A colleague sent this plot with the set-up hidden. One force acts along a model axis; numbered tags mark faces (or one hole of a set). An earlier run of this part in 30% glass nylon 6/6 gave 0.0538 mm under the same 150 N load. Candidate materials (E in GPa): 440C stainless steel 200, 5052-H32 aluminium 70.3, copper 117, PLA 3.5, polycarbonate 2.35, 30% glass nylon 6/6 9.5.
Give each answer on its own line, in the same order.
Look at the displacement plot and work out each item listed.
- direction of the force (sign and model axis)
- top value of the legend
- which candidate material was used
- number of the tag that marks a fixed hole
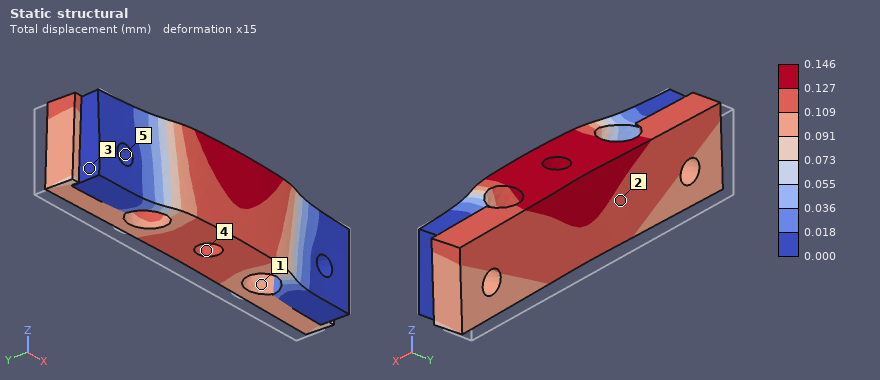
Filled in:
-Y
0.146 mm
PLA
5
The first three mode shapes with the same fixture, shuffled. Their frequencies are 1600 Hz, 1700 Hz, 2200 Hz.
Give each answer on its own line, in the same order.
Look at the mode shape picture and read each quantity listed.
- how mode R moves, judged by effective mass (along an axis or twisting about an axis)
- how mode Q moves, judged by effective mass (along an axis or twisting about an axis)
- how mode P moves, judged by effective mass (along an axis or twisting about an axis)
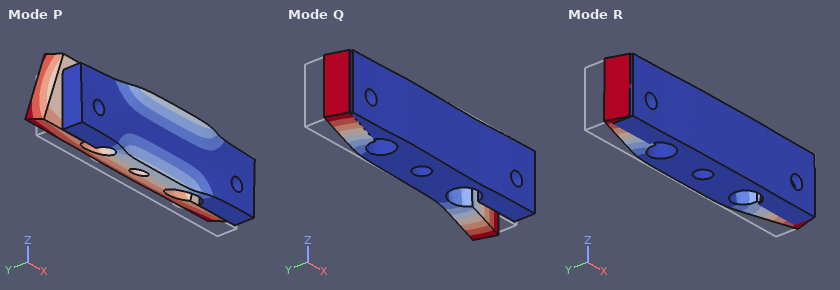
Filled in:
along Y
twisting about Z
along Z
